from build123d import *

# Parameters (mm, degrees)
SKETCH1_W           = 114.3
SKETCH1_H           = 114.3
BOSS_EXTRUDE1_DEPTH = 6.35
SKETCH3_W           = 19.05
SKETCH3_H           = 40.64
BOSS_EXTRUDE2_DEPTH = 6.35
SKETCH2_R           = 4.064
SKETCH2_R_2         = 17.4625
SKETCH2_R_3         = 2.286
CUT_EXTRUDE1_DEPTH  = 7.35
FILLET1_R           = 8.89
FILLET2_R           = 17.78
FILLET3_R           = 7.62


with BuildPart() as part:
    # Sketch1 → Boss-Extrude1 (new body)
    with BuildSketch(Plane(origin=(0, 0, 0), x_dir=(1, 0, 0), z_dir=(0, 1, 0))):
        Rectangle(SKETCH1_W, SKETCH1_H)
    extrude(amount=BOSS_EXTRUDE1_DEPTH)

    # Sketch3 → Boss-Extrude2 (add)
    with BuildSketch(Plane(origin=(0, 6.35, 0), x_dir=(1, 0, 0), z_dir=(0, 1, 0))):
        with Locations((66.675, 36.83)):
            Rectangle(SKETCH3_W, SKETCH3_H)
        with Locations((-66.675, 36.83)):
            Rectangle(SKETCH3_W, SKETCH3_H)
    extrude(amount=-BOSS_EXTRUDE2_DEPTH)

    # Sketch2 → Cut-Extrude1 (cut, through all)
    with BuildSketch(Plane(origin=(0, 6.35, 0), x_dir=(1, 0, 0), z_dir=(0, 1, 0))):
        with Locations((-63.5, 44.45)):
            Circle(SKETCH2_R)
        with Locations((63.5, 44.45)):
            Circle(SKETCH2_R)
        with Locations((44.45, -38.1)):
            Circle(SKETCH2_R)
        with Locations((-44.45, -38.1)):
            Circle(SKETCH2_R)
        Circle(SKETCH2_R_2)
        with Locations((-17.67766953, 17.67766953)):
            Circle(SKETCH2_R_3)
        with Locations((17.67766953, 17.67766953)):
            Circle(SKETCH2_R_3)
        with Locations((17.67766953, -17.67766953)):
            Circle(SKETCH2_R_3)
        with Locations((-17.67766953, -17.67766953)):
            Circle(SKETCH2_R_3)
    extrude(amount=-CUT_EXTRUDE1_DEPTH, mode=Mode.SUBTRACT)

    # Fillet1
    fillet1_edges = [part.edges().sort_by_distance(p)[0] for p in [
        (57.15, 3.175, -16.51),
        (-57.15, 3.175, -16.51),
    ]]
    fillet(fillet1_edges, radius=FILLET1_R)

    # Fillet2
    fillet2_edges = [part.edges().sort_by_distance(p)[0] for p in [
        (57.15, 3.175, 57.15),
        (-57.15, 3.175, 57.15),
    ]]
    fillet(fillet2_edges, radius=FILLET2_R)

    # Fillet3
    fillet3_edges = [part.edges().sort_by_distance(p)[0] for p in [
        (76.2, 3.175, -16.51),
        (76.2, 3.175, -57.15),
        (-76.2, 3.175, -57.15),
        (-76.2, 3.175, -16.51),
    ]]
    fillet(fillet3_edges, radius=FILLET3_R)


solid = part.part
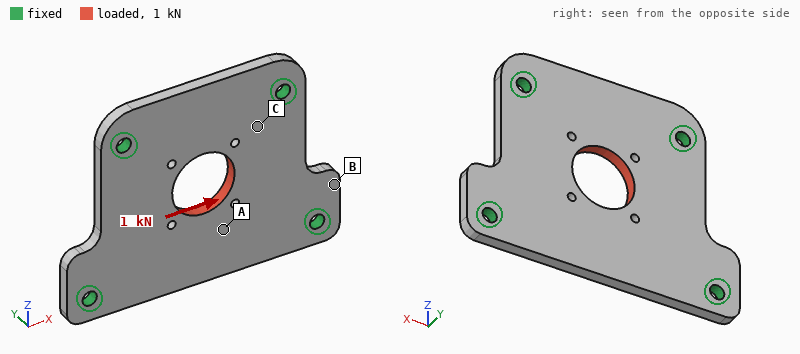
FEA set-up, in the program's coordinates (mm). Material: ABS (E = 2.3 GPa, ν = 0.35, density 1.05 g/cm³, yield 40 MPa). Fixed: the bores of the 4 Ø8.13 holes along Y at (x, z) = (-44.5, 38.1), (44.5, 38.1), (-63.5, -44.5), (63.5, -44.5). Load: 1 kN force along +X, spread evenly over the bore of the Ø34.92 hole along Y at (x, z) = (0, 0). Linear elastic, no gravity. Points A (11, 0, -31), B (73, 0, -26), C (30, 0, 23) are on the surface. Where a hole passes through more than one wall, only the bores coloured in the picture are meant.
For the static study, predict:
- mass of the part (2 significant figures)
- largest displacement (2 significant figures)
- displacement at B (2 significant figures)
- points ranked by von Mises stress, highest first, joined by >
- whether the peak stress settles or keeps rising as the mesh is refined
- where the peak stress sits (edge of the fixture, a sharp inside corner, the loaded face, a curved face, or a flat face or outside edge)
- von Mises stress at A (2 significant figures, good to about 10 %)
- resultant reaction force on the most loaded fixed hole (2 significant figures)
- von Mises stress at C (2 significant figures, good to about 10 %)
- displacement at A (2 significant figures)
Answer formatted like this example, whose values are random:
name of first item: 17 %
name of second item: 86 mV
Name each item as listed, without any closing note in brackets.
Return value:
mass of the part: 88 g
largest displacement: 42 µm
displacement at B: 19 µm
points ranked by von Mises stress, highest first, joined by >: C > A > B
whether the peak stress settles or keeps rising as the mesh is refined: keeps rising
where the peak stress sits: edge of the fixture
von Mises stress at A: 0.84 MPa
resultant reaction force on the most loaded fixed hole: 280 N
von Mises stress at C: 1.5 MPa
displacement at A: 25 µm
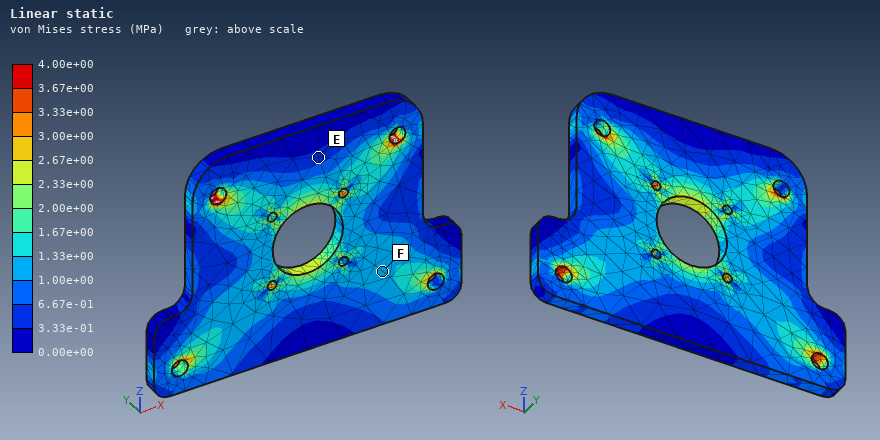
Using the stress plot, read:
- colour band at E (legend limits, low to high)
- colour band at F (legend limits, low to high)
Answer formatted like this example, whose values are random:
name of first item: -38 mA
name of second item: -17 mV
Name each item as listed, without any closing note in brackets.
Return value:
colour band at E: 3.33e-01 to 6.67e-01 MPa
colour band at F: 1.00e+00 to 1.33e+00 MPa
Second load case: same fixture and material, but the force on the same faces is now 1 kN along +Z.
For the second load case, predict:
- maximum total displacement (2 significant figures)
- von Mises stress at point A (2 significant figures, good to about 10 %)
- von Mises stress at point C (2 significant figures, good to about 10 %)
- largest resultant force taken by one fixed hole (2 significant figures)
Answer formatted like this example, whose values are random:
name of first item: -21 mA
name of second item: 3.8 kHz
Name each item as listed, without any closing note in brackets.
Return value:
maximum total displacement: 61 µm
von Mises stress at point A: 1.0 MPa
von Mises stress at point C: 2.0 MPa
largest resultant force taken by one fixed hole: 370 N
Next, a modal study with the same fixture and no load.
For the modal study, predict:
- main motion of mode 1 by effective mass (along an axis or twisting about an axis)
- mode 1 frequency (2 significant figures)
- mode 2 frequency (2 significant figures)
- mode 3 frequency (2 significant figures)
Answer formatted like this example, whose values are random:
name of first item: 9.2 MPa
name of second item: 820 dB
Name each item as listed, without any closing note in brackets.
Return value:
main motion of mode 1 by effective mass: along Y
mode 1 frequency: 630 Hz
mode 2 frequency: 1100 Hz
mode 3 frequency: 1300 Hz
